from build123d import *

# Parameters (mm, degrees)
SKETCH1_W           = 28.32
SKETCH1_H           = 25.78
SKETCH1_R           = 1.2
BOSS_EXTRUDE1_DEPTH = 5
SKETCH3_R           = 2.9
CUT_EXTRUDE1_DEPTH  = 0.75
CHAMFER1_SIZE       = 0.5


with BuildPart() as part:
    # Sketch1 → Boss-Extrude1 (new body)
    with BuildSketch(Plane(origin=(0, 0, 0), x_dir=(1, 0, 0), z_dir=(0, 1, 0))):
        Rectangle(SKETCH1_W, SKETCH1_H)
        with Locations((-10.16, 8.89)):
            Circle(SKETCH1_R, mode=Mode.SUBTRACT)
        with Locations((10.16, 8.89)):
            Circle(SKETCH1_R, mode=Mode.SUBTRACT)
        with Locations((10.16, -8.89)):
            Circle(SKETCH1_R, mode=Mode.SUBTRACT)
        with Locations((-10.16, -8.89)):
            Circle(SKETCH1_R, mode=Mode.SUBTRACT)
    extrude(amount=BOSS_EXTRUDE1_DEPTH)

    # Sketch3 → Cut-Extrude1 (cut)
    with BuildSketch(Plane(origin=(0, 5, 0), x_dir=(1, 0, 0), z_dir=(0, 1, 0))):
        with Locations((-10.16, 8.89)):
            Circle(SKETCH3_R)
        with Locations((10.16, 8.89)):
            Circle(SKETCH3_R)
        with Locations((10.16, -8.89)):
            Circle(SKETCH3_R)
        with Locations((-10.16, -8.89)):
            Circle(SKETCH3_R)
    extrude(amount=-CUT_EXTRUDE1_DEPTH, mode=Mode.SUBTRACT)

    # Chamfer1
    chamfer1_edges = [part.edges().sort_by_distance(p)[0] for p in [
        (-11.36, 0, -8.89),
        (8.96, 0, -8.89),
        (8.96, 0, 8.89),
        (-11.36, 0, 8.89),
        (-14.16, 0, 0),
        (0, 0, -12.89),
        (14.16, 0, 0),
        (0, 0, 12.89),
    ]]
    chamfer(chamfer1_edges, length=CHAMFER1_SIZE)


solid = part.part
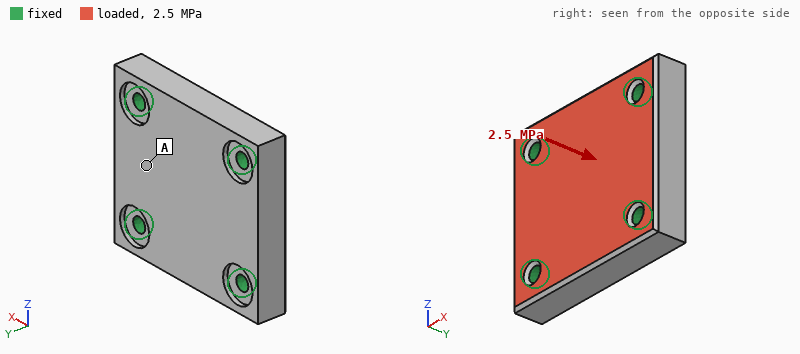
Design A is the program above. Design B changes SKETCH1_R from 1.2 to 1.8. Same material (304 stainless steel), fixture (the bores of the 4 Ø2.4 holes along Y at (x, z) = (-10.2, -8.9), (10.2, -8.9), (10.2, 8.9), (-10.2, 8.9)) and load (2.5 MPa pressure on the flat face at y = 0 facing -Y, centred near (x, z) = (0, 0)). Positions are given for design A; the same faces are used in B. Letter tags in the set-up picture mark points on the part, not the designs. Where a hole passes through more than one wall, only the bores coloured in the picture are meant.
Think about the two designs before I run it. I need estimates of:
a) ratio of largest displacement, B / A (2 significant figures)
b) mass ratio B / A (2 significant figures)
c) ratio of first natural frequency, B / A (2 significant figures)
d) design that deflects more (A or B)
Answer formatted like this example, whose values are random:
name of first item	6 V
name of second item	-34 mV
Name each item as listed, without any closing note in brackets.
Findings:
ratio of largest displacement, B / A	0.78
mass ratio B / A	0.97
ratio of first natural frequency, B / A	1.1
design that deflects more	A
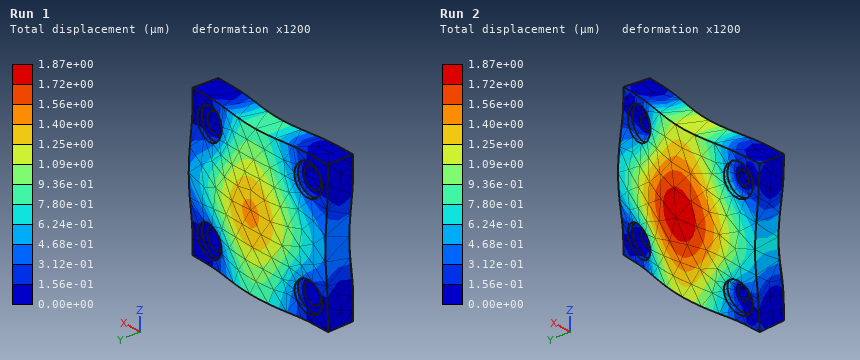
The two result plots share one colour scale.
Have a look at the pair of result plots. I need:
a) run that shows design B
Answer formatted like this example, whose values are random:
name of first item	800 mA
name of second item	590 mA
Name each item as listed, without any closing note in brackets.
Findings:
run that shows design B	Run 1
